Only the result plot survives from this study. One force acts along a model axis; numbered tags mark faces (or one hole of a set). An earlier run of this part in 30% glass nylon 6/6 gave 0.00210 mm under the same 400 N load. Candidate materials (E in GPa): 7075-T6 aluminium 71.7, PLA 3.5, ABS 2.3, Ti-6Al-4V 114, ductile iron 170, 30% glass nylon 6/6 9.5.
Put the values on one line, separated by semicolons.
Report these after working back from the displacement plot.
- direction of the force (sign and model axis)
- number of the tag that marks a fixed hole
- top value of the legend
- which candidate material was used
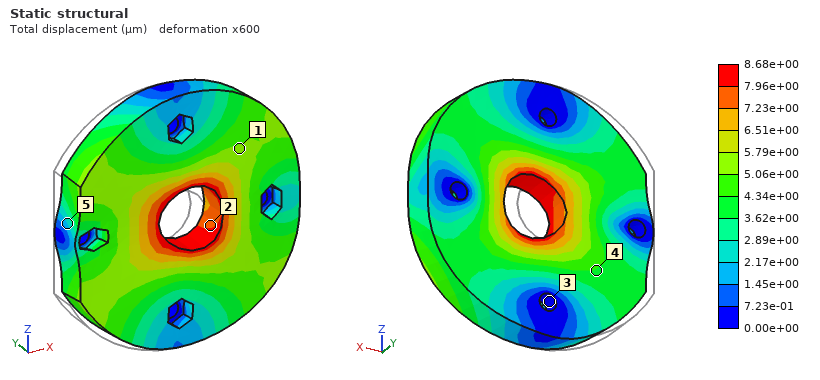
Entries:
+X; 3; 8.68e+00 µm; ABS
